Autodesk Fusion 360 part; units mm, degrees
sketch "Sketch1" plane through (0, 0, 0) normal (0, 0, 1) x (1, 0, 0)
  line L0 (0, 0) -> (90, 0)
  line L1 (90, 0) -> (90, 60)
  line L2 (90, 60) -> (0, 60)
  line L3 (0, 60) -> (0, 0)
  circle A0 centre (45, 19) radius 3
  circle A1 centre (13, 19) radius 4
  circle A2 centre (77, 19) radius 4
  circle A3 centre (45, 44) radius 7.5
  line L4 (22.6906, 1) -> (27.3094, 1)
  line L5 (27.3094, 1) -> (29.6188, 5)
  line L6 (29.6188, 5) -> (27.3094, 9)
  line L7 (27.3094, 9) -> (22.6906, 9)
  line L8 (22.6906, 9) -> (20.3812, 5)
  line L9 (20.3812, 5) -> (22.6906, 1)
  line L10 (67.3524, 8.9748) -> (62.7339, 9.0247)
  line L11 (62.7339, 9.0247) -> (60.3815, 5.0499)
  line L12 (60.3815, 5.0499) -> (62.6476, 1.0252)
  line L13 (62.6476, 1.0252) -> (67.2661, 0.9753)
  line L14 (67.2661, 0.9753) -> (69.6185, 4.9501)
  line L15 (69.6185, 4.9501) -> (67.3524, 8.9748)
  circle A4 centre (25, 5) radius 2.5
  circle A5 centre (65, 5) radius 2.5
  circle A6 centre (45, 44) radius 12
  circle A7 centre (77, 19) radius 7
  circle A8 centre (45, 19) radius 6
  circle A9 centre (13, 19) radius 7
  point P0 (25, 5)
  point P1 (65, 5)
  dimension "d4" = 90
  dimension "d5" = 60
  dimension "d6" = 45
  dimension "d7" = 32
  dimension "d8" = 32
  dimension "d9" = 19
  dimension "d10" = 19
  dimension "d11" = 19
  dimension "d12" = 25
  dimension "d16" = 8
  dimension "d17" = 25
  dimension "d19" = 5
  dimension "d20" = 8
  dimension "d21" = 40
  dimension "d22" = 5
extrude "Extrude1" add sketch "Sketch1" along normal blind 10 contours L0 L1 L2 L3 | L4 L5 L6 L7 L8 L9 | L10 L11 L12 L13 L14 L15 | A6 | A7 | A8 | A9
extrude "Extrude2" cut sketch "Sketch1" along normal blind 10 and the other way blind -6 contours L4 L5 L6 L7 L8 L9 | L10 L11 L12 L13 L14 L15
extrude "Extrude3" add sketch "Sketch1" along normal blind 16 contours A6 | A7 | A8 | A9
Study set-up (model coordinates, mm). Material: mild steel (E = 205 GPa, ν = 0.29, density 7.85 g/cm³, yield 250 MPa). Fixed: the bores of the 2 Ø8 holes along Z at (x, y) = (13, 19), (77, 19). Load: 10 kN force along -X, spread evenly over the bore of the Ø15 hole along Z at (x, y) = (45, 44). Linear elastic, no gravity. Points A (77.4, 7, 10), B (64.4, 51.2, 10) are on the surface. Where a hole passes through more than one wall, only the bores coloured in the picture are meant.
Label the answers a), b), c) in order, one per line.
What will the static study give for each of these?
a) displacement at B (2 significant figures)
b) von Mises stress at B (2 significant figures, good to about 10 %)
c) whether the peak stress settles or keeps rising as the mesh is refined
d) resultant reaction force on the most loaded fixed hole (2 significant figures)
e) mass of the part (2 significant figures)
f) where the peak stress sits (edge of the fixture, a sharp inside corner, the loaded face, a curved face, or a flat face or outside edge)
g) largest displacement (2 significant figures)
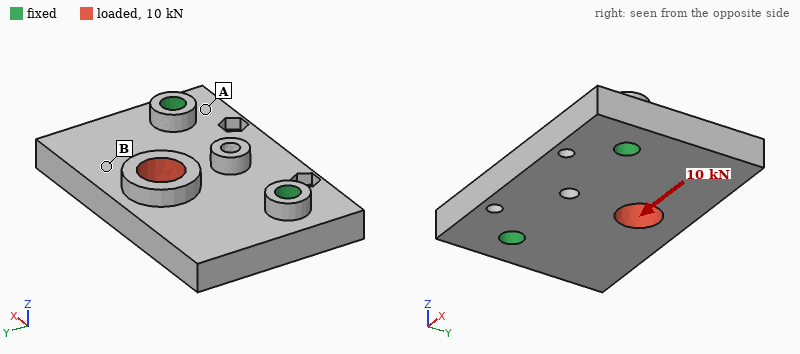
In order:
a) 7.0 µm
b) 21 MPa
c) keeps rising
d) 6.1 kN
e) 420 g
f) edge of the fixture
g) 11 µm
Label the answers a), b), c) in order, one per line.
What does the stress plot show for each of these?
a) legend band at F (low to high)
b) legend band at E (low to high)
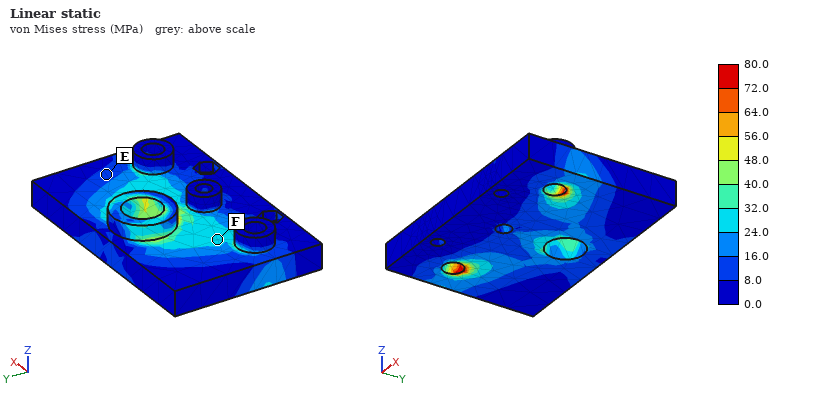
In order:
a) 24.0 to 32.0 MPa
b) 8.0 to 16.0 MPa
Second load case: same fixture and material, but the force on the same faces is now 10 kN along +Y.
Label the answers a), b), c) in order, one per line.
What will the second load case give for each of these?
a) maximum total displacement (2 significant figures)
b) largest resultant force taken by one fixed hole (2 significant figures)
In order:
a) 22 µm
b) 5.3 kN
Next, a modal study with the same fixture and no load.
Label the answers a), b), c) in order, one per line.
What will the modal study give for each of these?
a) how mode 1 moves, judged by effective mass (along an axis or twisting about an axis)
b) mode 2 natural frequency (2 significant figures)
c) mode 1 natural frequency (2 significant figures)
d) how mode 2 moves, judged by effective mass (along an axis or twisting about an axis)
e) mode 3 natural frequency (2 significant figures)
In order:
a) along Z
b) 7000 Hz
c) 4300 Hz
d) twisting about Y
e) 10 kHz
